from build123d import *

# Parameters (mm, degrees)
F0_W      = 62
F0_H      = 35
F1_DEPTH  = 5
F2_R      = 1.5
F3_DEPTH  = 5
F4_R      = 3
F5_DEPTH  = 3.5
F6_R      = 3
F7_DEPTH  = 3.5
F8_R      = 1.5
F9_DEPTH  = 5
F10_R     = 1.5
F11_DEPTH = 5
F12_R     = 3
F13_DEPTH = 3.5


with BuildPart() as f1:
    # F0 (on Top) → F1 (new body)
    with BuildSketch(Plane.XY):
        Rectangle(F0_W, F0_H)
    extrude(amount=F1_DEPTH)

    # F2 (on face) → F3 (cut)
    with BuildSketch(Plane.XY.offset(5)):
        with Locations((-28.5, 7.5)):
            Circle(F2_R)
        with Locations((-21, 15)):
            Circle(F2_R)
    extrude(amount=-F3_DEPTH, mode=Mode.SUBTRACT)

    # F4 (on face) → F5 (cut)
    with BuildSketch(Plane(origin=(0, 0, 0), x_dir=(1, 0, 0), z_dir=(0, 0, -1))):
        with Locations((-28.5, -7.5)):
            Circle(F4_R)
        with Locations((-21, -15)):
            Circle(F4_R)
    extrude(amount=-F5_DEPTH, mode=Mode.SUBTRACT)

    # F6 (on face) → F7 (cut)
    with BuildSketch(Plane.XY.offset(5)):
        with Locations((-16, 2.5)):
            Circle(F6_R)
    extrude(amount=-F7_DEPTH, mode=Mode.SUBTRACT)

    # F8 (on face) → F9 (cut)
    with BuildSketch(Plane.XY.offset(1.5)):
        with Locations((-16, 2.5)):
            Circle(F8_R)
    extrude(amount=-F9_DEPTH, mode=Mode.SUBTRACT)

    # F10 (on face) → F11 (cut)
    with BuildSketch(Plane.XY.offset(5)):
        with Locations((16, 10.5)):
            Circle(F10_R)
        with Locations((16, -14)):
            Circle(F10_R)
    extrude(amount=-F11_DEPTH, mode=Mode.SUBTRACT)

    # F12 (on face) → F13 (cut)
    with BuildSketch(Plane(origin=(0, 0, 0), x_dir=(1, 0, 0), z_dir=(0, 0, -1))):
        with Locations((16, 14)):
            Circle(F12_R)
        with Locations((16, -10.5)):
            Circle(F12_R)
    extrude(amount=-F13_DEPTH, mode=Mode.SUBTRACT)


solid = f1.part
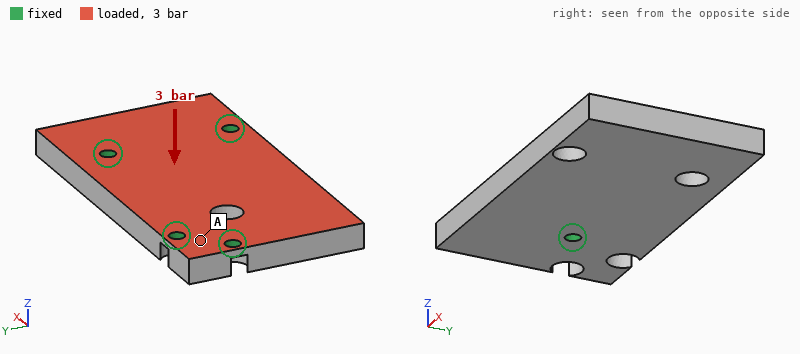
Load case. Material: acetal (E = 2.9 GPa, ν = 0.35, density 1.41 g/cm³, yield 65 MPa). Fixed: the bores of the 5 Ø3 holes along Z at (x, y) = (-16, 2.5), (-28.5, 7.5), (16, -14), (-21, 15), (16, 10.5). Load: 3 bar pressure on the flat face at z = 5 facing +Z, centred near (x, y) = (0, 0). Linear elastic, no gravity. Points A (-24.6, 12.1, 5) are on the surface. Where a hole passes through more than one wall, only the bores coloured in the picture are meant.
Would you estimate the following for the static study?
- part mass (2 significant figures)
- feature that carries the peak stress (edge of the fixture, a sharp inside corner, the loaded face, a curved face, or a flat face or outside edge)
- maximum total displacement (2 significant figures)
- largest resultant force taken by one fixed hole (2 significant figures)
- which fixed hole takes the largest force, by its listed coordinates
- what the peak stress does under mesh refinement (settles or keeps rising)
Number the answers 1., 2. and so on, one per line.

1. 15 g
2. edge of the fixture
3. 0.40 mm
4. 270 N
5. (-16, 2.5)
6. keeps rising
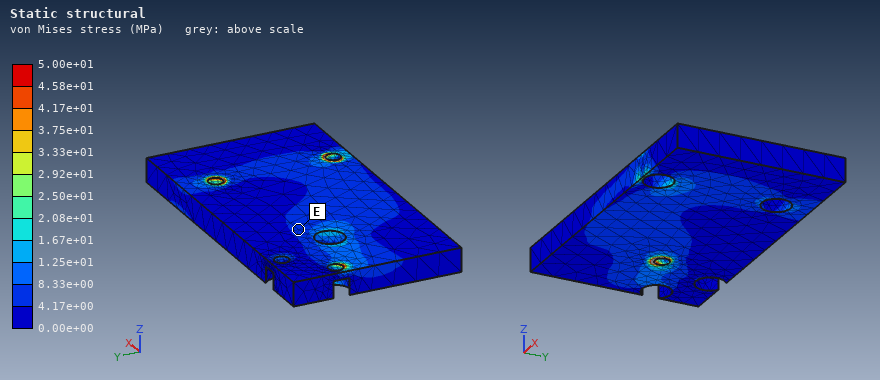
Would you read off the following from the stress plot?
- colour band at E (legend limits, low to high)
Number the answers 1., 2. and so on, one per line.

1. 4.17e+00 to 8.33e+00 MPa
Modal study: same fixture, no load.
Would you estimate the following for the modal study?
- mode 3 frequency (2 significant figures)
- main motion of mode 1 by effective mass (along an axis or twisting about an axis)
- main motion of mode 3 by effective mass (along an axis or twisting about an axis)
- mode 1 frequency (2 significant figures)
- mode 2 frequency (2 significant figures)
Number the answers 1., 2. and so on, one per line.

1. 3700 Hz
2. along Z
3. along Z
4. 2100 Hz
5. 2500 Hz
